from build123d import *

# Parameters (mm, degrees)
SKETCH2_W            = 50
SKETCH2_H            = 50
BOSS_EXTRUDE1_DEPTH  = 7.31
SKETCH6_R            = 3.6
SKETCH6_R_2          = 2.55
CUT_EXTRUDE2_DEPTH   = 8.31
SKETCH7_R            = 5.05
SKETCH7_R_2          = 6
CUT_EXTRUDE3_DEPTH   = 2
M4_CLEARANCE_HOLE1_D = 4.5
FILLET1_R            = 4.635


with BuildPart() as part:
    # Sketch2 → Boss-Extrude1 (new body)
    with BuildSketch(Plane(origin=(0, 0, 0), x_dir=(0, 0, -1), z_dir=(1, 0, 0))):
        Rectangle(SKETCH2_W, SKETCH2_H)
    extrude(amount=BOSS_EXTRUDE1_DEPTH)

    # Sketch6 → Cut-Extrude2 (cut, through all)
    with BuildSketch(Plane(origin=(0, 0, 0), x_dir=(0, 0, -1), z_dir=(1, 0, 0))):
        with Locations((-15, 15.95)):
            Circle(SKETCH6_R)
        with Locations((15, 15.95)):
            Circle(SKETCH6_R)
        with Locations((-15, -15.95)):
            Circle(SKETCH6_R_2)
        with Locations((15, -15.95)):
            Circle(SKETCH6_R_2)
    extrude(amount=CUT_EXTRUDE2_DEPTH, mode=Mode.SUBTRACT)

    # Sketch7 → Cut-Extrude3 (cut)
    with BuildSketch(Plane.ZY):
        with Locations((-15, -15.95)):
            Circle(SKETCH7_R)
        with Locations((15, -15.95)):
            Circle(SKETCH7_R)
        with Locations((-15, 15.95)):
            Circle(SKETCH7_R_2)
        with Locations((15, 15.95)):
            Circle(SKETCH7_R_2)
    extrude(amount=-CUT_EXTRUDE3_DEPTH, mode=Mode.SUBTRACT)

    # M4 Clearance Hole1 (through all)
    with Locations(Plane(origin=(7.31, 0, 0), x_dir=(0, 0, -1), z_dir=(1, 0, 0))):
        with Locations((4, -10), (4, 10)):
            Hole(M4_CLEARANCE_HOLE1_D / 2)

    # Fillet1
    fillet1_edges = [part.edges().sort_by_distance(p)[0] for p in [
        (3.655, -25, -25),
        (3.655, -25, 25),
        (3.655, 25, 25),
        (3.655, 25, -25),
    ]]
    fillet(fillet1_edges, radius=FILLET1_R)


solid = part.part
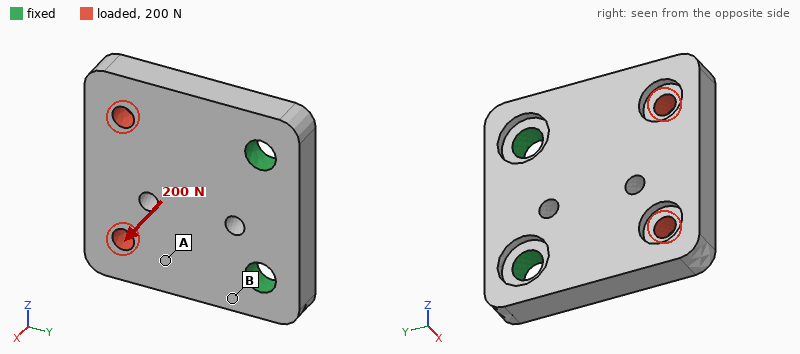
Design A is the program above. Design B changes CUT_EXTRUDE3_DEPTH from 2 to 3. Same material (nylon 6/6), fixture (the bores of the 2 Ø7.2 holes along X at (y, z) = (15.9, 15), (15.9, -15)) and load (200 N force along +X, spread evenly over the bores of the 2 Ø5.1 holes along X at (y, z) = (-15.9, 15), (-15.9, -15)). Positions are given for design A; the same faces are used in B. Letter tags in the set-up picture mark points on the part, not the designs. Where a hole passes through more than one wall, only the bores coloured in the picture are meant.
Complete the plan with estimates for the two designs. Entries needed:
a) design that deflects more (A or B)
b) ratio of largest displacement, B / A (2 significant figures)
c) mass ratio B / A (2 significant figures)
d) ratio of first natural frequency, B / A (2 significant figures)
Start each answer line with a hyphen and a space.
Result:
- B
- 1.2
- 0.98
- 0.91
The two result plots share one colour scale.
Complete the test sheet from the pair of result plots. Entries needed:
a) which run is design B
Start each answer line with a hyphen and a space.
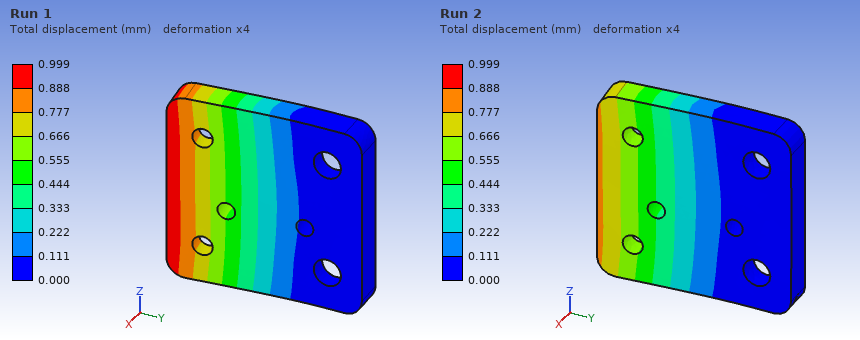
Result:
- Run 1
